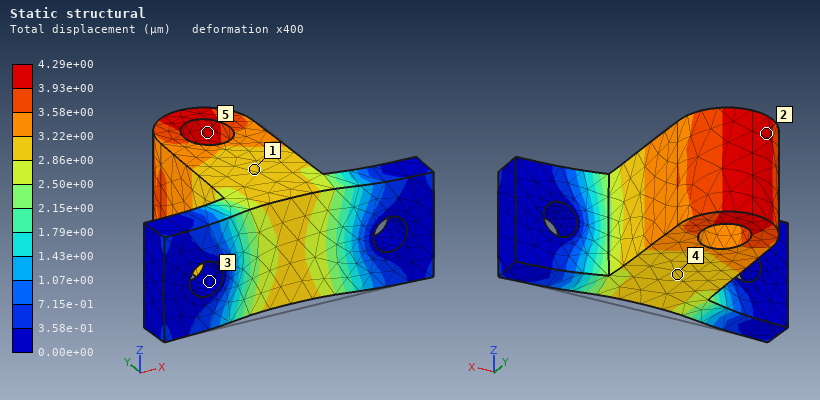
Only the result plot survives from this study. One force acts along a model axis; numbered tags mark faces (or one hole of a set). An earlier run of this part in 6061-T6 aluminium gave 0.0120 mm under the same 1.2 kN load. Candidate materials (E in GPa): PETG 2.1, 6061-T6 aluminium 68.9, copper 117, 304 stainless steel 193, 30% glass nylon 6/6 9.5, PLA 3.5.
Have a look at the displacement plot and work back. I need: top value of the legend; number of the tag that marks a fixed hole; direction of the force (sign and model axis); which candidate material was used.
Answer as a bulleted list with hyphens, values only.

- 4.29e+00 µm
- 3
- +Y
- 304 stainless steel
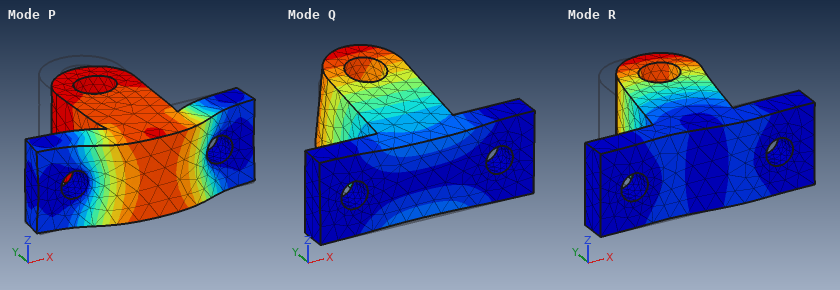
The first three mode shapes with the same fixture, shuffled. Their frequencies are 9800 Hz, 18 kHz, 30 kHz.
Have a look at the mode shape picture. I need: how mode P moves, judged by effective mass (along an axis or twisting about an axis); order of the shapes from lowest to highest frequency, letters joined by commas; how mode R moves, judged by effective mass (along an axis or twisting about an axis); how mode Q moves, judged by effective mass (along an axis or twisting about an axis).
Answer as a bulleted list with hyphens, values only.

- along Y
- Q, R, P
- along X
- along Z
